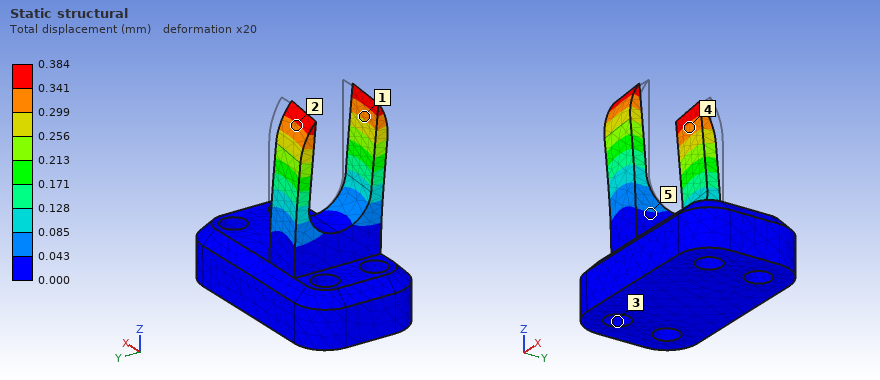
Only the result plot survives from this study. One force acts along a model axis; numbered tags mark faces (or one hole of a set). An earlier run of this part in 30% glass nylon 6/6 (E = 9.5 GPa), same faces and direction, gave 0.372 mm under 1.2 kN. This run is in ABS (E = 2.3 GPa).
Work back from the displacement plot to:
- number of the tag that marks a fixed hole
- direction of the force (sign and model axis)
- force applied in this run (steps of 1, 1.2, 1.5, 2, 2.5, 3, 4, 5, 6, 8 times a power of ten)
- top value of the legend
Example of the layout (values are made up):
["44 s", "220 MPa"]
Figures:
["3", "-X", "300 N", "0.384 mm"]
